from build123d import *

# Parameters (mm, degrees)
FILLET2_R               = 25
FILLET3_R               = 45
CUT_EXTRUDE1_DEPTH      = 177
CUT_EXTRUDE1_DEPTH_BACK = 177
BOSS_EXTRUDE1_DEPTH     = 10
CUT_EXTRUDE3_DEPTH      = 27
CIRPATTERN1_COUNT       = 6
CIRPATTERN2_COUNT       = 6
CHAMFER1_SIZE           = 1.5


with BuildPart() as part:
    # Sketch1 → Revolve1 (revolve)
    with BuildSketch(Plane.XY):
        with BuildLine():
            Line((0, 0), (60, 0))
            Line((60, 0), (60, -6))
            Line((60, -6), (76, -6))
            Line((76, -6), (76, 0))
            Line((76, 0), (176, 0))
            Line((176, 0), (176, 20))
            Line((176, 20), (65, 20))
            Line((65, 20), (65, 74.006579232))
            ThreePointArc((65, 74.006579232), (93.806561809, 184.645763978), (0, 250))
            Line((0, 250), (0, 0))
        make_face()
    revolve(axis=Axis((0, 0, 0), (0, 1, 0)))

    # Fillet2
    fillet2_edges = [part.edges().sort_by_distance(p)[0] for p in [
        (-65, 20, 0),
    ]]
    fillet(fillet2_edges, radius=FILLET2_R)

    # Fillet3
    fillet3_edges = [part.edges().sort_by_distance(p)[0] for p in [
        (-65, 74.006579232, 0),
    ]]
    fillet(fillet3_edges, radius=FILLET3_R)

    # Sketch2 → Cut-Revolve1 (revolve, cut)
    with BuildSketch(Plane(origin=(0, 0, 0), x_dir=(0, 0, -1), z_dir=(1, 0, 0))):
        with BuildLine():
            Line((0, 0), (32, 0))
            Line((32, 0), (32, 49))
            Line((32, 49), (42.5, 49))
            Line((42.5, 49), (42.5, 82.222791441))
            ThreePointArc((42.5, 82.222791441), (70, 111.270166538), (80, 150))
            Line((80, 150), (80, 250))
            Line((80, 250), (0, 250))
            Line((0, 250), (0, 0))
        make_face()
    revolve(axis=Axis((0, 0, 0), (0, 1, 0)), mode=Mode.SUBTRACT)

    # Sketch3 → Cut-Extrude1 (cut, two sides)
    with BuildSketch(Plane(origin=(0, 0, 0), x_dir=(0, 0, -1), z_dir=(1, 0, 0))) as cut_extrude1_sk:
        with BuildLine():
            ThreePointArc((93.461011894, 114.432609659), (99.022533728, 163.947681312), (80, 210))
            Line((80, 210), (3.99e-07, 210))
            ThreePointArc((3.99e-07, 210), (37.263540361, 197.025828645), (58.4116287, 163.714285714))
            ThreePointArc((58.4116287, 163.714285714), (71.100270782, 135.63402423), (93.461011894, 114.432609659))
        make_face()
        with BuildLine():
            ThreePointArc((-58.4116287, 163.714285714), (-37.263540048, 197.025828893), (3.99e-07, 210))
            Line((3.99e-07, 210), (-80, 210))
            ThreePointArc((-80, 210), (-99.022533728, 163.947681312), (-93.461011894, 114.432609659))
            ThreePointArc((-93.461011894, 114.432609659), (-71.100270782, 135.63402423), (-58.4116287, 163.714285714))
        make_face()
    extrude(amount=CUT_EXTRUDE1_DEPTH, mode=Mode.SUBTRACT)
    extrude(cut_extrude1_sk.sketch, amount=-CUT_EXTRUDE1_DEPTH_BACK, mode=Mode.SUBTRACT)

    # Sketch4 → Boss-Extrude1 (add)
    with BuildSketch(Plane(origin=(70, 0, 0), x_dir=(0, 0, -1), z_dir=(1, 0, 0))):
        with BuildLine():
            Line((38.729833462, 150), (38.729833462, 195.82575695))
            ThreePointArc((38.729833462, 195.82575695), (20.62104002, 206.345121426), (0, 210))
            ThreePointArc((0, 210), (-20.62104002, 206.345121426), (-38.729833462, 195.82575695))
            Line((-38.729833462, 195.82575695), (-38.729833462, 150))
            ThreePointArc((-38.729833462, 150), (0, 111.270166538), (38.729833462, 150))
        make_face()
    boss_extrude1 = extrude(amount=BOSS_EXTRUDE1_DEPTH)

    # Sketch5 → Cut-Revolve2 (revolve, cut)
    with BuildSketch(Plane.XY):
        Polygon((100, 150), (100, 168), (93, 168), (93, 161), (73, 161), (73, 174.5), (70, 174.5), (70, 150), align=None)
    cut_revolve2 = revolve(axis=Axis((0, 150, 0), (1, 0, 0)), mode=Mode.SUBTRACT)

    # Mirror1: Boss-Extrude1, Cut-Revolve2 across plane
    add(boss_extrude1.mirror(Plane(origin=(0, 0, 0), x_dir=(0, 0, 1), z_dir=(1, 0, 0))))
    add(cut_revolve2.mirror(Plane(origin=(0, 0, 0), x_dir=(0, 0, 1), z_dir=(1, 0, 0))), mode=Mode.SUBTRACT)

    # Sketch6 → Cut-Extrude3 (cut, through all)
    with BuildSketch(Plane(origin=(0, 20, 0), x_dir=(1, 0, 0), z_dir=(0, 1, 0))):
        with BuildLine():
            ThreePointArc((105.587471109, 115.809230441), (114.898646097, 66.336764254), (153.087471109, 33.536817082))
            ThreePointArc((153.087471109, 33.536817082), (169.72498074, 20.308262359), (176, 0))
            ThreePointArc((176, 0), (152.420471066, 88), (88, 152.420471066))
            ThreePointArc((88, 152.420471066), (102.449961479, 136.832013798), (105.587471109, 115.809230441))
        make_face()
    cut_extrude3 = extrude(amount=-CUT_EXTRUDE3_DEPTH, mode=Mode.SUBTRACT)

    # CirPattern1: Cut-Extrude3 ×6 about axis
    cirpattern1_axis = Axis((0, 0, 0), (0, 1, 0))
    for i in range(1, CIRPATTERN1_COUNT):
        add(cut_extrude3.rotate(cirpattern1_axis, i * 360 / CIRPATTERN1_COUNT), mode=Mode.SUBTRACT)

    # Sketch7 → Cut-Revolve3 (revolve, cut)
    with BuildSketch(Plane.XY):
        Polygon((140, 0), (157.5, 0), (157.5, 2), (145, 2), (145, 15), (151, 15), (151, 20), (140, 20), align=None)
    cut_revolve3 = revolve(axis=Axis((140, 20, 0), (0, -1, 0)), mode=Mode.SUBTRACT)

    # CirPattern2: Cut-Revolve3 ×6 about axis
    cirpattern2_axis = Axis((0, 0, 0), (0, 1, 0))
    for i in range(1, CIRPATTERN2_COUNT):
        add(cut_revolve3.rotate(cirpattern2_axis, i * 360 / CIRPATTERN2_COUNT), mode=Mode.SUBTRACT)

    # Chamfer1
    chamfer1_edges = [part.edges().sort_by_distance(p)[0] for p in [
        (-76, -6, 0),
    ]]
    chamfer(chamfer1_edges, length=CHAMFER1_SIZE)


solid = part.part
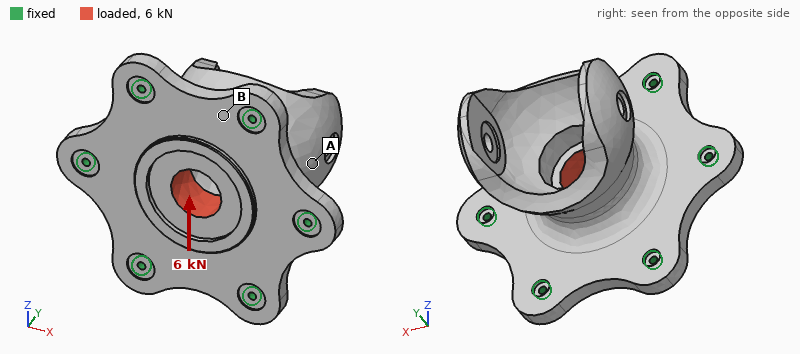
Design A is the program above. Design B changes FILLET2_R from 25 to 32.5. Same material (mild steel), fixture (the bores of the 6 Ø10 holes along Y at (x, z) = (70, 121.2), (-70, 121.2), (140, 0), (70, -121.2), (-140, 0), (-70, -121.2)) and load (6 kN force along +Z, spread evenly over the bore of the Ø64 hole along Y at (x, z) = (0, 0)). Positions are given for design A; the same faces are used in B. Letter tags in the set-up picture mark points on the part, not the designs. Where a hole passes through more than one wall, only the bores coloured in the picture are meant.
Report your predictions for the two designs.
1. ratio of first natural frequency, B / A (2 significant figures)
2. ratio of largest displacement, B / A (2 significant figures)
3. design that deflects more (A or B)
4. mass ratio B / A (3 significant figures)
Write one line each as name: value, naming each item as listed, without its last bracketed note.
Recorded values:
ratio of first natural frequency, B / A: 1.1
ratio of largest displacement, B / A: 0.83
design that deflects more: A
mass ratio B / A: 1.01
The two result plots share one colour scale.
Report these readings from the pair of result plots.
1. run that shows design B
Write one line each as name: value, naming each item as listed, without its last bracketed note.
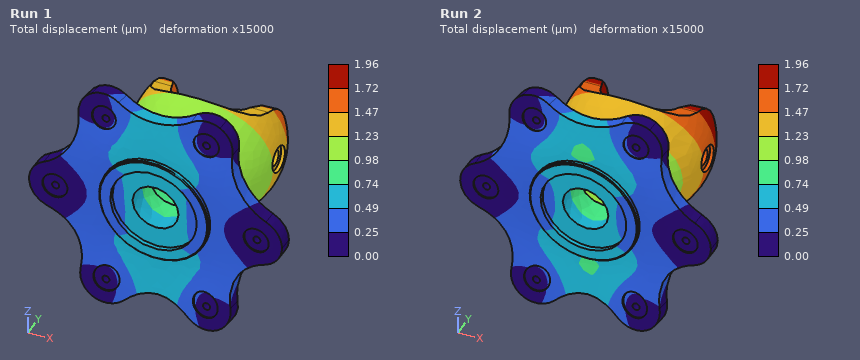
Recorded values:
run that shows design B: Run 1
